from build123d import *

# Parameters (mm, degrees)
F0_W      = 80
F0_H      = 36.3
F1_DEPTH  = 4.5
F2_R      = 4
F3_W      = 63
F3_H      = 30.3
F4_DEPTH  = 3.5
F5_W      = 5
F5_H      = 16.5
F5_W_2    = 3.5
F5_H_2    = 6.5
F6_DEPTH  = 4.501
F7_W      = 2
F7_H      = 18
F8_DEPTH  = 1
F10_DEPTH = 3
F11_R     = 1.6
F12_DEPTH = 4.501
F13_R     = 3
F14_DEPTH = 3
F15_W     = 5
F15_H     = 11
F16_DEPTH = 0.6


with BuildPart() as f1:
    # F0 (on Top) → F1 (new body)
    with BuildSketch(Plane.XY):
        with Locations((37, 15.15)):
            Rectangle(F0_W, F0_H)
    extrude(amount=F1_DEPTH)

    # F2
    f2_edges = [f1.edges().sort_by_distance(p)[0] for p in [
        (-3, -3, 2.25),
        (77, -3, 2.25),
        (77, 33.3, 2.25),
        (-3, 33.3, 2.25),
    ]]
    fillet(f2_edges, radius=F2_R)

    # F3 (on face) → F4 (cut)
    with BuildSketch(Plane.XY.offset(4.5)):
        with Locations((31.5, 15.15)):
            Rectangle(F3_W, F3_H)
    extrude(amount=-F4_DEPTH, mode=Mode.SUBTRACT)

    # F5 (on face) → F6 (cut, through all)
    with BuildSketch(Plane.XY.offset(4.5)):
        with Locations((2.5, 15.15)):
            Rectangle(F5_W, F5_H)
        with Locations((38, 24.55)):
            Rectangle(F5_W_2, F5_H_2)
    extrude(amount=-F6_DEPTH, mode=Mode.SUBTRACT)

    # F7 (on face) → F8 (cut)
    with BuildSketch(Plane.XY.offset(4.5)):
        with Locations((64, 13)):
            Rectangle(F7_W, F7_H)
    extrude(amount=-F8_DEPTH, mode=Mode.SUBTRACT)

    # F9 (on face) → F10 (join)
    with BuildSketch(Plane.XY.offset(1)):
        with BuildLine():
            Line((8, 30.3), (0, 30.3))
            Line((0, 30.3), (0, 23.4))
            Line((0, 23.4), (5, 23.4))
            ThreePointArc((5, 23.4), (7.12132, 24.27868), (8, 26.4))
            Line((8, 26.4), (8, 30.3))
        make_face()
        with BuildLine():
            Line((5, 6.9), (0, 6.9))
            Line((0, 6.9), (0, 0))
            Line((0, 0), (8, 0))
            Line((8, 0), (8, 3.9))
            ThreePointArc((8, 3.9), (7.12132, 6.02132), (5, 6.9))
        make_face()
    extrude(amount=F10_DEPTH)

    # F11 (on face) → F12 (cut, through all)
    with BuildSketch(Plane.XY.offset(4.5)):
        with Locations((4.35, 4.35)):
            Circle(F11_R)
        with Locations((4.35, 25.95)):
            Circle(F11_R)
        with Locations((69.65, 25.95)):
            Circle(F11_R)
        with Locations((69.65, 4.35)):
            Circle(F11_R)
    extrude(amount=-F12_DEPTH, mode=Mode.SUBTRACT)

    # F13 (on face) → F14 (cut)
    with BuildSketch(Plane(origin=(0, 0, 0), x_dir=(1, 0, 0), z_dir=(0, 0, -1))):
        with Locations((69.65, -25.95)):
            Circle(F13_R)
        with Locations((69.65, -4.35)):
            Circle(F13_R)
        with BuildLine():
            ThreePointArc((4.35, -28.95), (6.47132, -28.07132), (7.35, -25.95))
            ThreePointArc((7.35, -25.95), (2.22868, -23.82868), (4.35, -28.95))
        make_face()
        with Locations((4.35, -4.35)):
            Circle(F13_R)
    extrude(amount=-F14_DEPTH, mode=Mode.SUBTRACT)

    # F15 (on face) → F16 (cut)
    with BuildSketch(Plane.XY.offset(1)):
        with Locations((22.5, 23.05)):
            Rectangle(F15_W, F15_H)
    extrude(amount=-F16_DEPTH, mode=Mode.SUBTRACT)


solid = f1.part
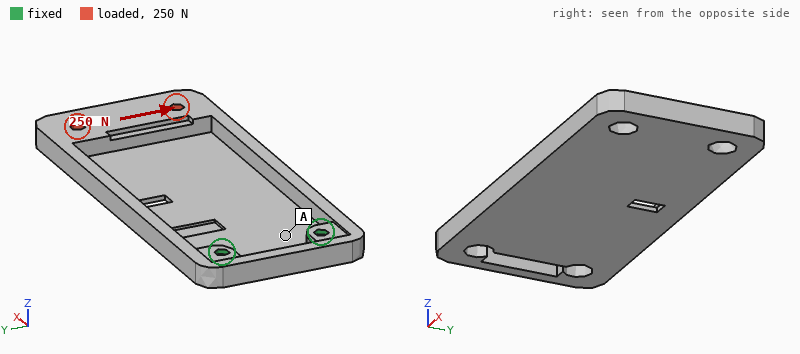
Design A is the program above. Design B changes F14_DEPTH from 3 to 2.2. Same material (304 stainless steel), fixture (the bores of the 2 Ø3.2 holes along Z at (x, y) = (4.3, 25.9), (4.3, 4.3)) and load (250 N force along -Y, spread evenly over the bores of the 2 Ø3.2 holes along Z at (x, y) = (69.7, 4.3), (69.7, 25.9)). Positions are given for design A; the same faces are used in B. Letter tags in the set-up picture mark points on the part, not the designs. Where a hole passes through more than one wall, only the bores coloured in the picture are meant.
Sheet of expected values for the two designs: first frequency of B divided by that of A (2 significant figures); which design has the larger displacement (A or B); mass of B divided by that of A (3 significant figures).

1.1
A
1.01
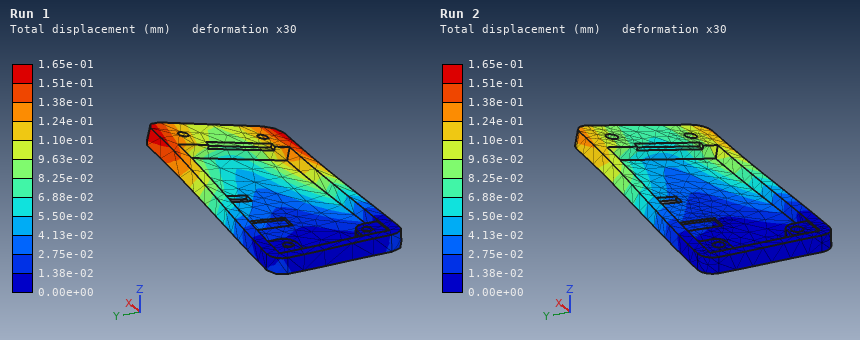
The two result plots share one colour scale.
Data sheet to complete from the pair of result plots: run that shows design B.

Run 2
